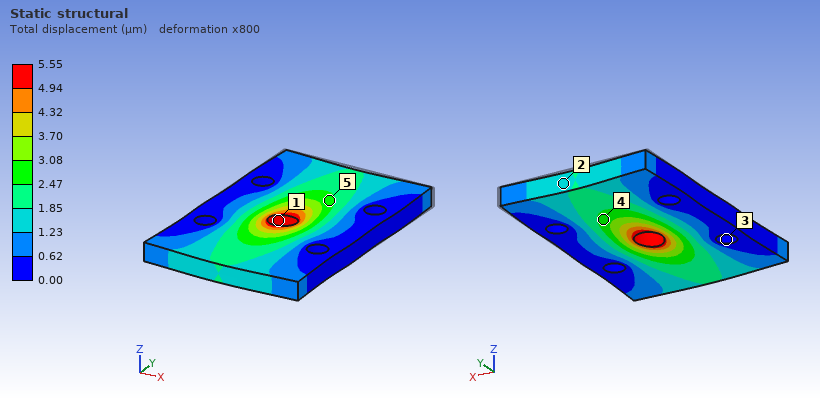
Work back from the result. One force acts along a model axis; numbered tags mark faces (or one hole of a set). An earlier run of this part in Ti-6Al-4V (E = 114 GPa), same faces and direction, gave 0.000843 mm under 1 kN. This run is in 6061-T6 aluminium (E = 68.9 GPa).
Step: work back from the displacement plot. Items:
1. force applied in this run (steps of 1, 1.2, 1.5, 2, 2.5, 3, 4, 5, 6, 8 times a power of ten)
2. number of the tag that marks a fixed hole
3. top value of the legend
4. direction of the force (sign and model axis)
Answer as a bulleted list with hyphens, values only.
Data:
- 4 kN
- 3
- 5.55 µm
- -Y
